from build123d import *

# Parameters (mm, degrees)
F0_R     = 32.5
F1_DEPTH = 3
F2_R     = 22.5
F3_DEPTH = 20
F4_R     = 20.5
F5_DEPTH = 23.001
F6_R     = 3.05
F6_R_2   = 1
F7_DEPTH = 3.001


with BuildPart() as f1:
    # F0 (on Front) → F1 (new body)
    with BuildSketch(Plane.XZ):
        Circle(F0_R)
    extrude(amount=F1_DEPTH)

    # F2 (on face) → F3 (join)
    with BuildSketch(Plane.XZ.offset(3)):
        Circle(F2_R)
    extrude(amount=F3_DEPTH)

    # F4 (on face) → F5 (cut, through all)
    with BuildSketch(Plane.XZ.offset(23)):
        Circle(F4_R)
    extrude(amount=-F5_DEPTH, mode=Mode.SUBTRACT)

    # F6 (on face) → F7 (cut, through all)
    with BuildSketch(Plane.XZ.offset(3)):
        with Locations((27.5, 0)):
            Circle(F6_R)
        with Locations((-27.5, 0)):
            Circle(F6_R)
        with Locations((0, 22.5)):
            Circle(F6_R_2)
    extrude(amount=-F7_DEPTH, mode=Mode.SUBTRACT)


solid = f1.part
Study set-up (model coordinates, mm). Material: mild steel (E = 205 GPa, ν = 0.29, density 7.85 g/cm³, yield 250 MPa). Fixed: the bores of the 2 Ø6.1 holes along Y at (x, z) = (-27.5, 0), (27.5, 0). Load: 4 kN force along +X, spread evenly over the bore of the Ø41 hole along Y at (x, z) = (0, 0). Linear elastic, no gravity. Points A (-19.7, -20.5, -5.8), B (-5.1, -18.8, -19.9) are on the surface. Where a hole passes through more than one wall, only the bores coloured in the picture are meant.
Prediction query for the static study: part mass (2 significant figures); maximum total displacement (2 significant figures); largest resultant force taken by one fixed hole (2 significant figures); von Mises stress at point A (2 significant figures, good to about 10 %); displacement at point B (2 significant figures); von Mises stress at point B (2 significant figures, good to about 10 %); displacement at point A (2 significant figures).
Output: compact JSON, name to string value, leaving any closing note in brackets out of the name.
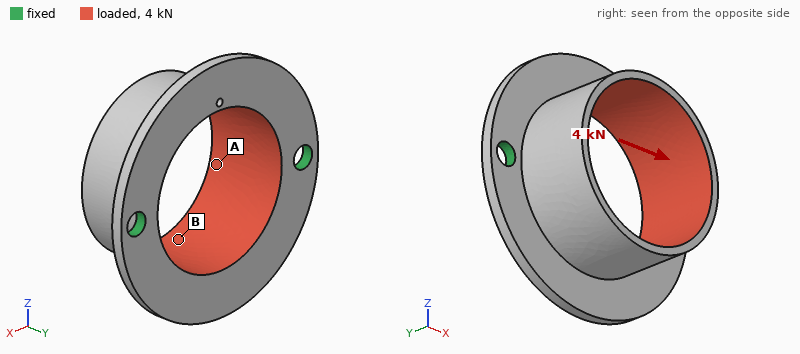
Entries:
{"part mass": "88 g", "maximum total displacement": "18 µm", "largest resultant force taken by one fixed hole": "2.2 kN", "von Mises stress at point A": "31 MPa", "displacement at point B": "16 µm", "von Mises stress at point B": "14 MPa", "displacement at point A": "11 µm"}
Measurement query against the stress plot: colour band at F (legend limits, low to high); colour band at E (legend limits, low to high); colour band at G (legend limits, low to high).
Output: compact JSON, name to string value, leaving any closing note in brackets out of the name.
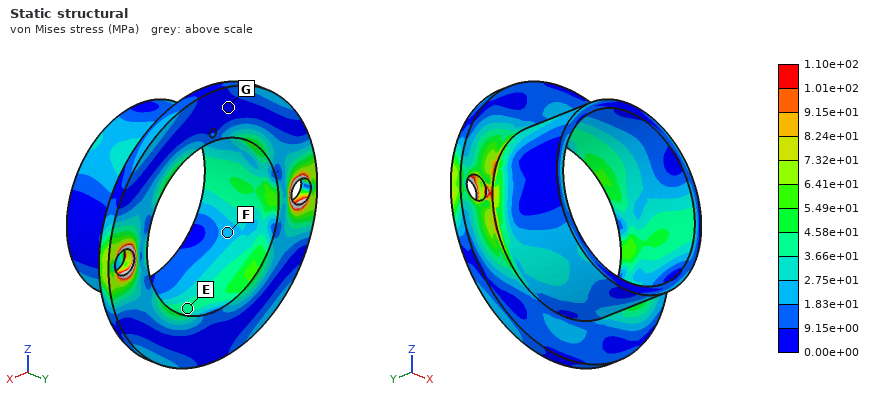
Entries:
{"colour band at F": "1.83e+01 to 2.75e+01 MPa", "colour band at E": "3.66e+01 to 4.58e+01 MPa", "colour band at G": "0.00e+00 to 9.15e+00 MPa"}
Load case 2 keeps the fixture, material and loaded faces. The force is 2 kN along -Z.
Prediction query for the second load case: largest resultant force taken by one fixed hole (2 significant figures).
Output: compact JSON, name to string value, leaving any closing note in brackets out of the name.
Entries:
{"largest resultant force taken by one fixed hole": "1.0 kN"}
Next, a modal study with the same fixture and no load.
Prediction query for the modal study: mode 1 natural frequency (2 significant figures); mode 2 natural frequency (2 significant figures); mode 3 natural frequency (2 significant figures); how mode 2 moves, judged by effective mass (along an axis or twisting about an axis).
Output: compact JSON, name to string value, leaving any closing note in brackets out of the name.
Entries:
{"mode 1 natural frequency": "2300 Hz", "mode 2 natural frequency": "3400 Hz", "mode 3 natural frequency": "5200 Hz", "how mode 2 moves, judged by effective mass": "along Y"}
